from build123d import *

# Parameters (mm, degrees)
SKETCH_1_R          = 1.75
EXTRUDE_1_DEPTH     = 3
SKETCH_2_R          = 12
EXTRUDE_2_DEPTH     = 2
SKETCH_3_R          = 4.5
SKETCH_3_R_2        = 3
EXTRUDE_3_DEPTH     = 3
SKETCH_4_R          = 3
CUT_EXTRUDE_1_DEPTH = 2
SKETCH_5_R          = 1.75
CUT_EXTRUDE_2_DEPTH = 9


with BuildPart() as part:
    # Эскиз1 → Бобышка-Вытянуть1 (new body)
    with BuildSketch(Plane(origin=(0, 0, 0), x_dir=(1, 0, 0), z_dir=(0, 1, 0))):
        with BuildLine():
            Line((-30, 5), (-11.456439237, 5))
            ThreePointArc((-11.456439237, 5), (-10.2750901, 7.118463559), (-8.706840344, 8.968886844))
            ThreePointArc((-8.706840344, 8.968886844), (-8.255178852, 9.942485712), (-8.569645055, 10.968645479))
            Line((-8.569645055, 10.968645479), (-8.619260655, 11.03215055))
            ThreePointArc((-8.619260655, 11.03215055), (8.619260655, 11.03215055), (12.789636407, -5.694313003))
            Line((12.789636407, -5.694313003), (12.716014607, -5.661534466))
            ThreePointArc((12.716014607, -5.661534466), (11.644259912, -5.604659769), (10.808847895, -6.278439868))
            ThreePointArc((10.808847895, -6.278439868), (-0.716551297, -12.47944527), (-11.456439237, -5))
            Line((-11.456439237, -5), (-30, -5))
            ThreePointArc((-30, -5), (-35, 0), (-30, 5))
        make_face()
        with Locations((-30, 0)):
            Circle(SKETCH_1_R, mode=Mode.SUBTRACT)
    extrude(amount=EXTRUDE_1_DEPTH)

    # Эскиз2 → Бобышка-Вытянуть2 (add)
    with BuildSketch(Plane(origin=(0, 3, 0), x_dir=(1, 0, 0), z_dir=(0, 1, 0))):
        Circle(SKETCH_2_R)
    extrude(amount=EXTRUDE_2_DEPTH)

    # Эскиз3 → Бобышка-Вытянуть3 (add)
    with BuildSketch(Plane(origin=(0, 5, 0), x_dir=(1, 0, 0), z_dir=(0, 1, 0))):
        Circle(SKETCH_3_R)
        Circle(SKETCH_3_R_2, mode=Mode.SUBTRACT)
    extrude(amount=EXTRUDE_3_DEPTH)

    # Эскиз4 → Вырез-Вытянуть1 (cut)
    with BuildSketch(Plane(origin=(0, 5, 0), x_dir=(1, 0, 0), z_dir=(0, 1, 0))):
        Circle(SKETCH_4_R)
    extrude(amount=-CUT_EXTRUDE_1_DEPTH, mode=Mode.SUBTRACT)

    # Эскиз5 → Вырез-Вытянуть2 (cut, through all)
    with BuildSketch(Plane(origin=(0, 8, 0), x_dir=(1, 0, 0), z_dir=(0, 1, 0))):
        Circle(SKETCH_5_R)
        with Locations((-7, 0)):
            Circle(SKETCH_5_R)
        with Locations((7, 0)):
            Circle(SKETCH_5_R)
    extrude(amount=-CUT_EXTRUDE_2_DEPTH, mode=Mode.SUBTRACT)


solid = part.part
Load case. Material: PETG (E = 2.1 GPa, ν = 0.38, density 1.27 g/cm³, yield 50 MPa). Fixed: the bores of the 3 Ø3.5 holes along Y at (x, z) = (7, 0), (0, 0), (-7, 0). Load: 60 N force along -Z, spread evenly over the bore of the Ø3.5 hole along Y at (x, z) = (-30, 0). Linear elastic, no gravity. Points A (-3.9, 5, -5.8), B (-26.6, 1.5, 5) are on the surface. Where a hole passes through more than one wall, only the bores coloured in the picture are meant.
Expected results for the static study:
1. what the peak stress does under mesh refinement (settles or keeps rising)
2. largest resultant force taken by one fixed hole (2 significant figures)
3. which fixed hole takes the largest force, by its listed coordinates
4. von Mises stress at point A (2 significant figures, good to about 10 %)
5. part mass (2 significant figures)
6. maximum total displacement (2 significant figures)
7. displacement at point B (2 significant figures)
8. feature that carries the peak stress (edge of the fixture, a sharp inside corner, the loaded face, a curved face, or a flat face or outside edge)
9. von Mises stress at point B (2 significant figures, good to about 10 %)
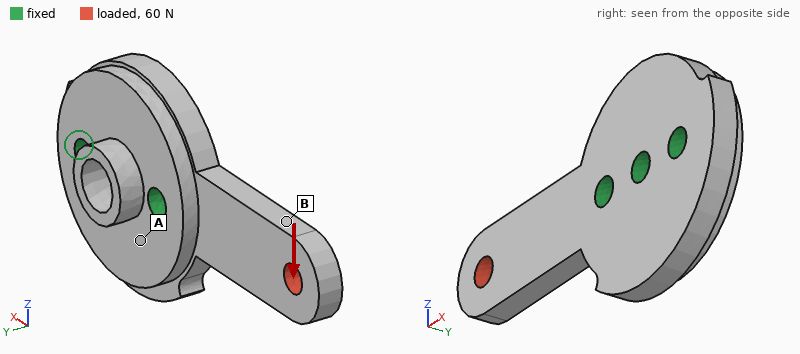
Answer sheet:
keeps rising
120 N
(-7, 0)
2.1 MPa
3.9 g
0.59 mm
0.37 mm
a sharp inside corner
5.1 MPa
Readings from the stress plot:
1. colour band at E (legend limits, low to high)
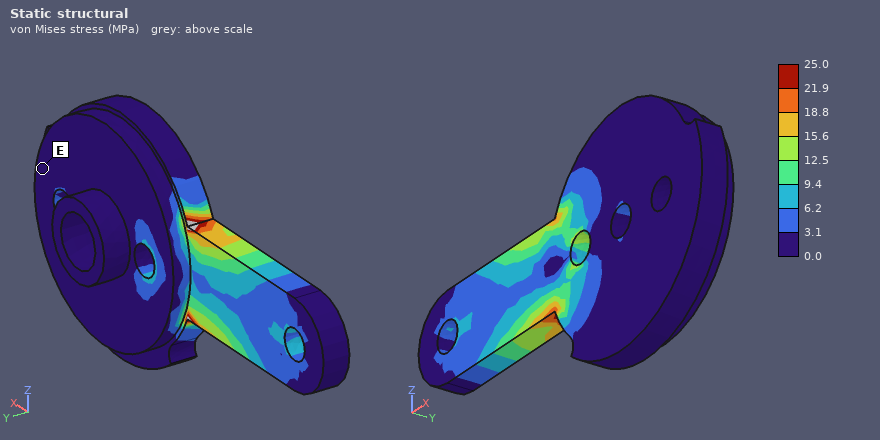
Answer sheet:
0.0 to 3.1 MPa
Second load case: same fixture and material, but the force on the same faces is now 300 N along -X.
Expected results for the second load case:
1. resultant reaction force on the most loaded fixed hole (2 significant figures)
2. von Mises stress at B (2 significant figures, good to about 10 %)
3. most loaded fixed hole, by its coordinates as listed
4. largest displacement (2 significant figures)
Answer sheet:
250 N
8.6 MPa
(-7, 0)
0.17 mm
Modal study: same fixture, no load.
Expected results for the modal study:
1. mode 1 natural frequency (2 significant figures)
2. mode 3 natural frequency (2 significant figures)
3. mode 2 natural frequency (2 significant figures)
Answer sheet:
1200 Hz
4700 Hz
3000 Hz
